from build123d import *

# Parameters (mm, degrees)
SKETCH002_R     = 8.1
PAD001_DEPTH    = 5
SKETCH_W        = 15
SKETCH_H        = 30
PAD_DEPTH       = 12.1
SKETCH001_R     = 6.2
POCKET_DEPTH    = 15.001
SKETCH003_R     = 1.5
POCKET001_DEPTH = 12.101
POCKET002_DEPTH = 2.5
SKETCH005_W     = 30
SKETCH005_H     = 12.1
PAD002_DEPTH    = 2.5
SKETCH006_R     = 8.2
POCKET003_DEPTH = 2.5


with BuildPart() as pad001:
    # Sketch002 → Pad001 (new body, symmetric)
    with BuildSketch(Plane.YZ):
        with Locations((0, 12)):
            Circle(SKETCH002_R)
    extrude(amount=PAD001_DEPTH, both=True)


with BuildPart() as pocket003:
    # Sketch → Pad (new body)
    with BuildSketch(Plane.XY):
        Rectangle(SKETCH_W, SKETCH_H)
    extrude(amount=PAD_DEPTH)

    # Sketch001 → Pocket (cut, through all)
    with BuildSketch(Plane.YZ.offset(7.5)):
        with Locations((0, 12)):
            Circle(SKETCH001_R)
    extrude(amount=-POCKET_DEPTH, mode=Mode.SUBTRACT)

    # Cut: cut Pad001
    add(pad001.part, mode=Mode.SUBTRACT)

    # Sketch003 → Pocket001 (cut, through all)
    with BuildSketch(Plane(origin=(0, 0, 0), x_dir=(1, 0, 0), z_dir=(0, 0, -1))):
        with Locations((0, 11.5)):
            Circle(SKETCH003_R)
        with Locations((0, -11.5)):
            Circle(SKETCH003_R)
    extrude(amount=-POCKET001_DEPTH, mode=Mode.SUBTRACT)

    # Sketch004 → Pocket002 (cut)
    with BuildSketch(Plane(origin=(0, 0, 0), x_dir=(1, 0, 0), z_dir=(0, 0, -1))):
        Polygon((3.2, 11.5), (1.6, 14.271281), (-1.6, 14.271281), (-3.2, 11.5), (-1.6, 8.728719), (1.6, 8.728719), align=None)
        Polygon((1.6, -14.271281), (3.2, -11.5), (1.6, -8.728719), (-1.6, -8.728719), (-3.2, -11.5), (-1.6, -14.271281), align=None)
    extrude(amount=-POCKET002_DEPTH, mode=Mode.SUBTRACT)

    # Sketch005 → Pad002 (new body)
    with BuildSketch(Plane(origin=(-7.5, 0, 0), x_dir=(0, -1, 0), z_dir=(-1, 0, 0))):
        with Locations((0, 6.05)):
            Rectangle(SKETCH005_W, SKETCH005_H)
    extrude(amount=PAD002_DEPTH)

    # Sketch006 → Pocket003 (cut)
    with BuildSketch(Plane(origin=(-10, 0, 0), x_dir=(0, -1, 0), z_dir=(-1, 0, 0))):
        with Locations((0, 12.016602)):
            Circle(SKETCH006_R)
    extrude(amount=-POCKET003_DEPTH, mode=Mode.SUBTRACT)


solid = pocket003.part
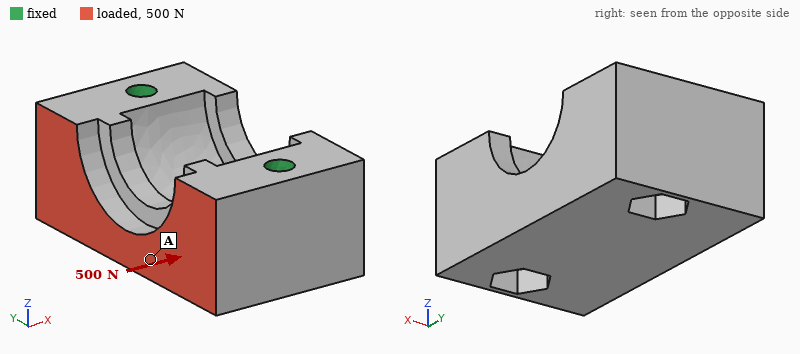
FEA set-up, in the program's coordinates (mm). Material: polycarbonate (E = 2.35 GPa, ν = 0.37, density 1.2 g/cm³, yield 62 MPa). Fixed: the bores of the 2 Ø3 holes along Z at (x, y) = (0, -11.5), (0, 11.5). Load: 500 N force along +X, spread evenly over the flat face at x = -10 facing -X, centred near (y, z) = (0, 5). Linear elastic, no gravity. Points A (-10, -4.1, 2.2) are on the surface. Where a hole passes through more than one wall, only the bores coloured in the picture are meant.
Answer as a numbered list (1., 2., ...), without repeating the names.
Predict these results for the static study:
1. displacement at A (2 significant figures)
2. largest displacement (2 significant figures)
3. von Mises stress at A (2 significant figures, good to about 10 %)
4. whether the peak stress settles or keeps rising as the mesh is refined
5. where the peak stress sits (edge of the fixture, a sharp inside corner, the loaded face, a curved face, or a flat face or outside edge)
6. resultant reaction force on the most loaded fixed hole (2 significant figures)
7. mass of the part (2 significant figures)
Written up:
1. 27 µm
2. 33 µm
3. 1.9 MPa
4. keeps rising
5. edge of the fixture
6. 250 N
7. 5.4 g
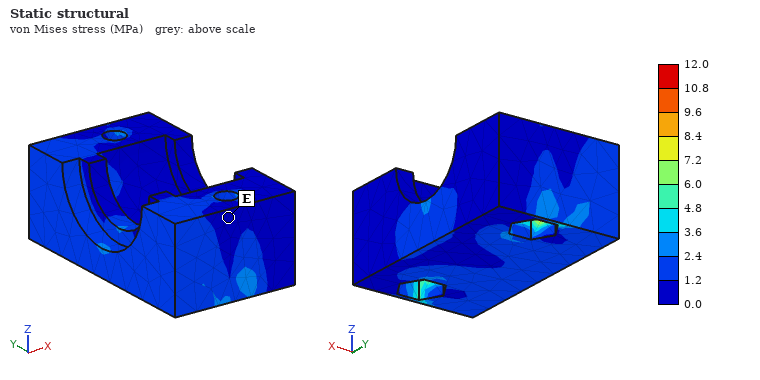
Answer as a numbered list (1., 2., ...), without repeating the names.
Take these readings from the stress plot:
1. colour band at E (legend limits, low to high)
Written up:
1. 0.0 to 1.2 MPa
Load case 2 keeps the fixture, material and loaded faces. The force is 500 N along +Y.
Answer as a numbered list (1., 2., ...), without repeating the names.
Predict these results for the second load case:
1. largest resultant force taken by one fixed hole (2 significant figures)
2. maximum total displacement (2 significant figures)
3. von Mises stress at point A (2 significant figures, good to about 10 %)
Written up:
1. 300 N
2. 71 µm
3. 5.1 MPa
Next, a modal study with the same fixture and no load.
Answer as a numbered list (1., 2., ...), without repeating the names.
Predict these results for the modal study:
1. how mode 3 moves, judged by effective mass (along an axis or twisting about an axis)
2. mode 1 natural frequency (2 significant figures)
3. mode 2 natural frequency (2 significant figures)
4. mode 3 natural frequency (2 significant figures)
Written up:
1. along Z
2. 9500 Hz
3. 12 kHz
4. 13 kHz
